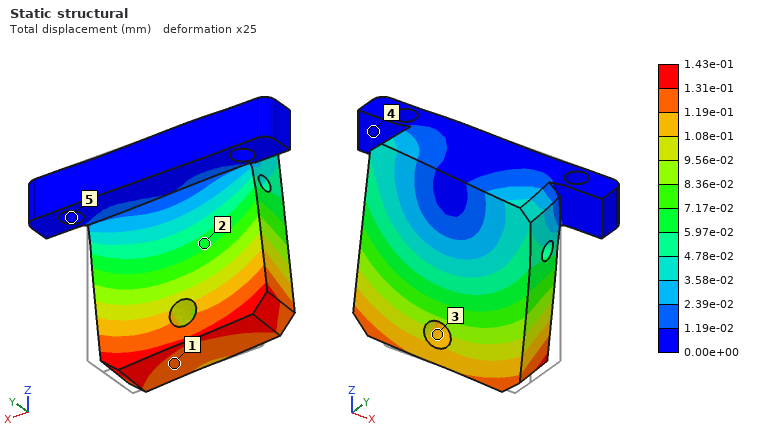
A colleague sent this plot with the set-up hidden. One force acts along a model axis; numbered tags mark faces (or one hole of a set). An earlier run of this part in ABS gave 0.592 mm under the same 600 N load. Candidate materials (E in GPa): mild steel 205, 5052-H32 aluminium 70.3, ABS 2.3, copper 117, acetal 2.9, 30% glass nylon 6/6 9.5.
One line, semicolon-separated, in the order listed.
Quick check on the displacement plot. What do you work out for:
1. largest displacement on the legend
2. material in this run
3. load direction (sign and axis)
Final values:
1.43e-01 mm; 30% glass nylon 6/6; -X
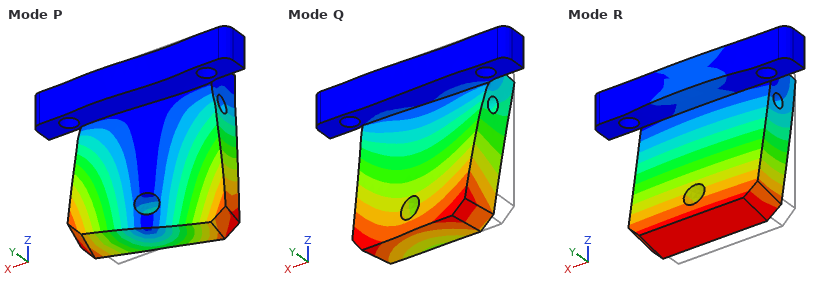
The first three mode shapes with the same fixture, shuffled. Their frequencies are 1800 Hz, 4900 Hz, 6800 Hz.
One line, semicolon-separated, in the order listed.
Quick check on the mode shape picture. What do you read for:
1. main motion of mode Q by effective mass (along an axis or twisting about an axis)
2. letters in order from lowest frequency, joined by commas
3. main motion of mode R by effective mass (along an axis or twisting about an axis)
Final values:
along X; R, Q, P; along Y
